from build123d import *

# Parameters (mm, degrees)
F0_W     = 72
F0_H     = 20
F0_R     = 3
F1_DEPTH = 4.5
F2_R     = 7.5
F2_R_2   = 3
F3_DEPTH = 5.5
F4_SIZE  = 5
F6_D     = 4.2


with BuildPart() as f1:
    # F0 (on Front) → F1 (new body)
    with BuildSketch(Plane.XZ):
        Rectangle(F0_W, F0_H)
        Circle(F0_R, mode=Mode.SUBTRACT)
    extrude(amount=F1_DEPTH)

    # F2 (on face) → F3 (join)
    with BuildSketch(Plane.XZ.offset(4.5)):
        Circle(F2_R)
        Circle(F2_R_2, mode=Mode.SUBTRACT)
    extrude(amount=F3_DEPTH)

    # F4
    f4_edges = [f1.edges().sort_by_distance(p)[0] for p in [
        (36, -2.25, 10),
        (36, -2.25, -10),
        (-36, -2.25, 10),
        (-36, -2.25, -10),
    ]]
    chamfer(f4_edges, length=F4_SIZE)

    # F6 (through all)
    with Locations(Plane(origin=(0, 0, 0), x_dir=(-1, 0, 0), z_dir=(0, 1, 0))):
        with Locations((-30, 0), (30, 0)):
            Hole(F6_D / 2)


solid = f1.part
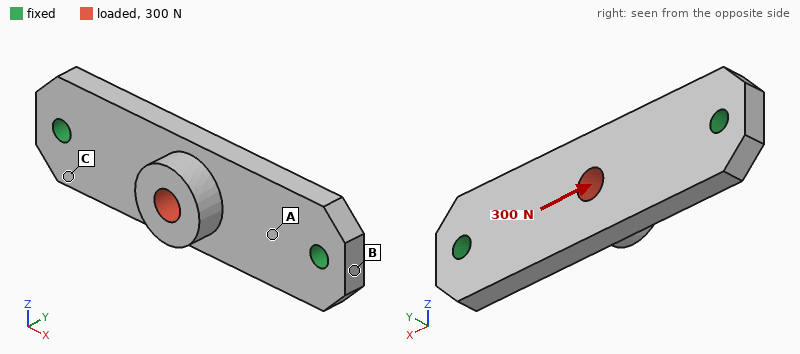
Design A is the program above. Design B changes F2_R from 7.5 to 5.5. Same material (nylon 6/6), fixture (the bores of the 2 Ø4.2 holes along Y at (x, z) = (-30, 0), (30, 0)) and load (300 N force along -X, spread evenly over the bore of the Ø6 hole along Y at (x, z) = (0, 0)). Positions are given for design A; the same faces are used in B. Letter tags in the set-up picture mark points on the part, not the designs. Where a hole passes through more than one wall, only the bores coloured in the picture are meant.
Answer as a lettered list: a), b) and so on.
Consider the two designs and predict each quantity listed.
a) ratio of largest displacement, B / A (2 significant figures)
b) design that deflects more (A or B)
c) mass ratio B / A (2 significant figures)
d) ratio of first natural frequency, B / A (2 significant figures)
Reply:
a) 1.4
b) B
c) 0.93
d) 1.0
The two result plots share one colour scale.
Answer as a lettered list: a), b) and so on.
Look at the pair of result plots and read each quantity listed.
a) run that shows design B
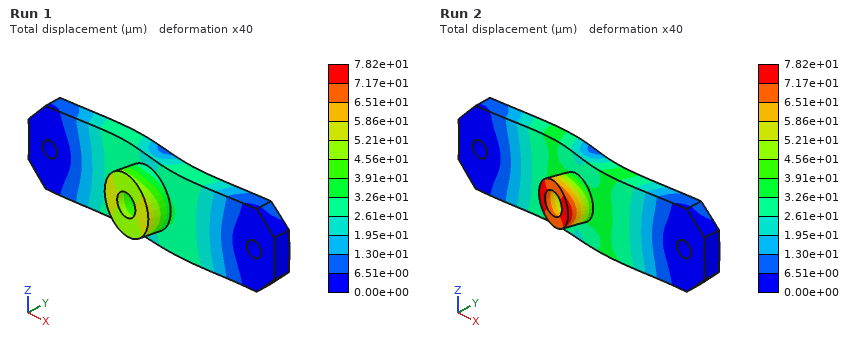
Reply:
a) Run 2
